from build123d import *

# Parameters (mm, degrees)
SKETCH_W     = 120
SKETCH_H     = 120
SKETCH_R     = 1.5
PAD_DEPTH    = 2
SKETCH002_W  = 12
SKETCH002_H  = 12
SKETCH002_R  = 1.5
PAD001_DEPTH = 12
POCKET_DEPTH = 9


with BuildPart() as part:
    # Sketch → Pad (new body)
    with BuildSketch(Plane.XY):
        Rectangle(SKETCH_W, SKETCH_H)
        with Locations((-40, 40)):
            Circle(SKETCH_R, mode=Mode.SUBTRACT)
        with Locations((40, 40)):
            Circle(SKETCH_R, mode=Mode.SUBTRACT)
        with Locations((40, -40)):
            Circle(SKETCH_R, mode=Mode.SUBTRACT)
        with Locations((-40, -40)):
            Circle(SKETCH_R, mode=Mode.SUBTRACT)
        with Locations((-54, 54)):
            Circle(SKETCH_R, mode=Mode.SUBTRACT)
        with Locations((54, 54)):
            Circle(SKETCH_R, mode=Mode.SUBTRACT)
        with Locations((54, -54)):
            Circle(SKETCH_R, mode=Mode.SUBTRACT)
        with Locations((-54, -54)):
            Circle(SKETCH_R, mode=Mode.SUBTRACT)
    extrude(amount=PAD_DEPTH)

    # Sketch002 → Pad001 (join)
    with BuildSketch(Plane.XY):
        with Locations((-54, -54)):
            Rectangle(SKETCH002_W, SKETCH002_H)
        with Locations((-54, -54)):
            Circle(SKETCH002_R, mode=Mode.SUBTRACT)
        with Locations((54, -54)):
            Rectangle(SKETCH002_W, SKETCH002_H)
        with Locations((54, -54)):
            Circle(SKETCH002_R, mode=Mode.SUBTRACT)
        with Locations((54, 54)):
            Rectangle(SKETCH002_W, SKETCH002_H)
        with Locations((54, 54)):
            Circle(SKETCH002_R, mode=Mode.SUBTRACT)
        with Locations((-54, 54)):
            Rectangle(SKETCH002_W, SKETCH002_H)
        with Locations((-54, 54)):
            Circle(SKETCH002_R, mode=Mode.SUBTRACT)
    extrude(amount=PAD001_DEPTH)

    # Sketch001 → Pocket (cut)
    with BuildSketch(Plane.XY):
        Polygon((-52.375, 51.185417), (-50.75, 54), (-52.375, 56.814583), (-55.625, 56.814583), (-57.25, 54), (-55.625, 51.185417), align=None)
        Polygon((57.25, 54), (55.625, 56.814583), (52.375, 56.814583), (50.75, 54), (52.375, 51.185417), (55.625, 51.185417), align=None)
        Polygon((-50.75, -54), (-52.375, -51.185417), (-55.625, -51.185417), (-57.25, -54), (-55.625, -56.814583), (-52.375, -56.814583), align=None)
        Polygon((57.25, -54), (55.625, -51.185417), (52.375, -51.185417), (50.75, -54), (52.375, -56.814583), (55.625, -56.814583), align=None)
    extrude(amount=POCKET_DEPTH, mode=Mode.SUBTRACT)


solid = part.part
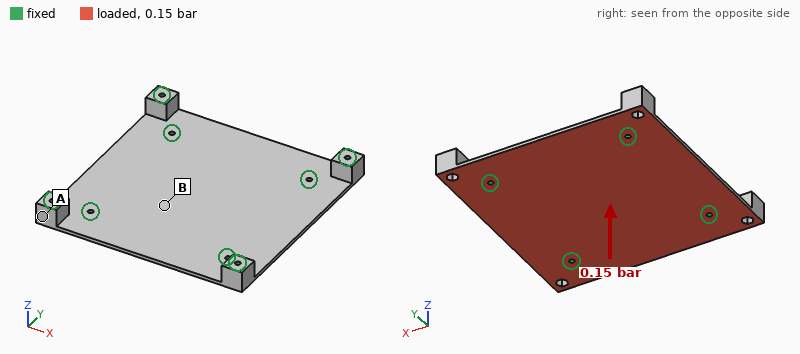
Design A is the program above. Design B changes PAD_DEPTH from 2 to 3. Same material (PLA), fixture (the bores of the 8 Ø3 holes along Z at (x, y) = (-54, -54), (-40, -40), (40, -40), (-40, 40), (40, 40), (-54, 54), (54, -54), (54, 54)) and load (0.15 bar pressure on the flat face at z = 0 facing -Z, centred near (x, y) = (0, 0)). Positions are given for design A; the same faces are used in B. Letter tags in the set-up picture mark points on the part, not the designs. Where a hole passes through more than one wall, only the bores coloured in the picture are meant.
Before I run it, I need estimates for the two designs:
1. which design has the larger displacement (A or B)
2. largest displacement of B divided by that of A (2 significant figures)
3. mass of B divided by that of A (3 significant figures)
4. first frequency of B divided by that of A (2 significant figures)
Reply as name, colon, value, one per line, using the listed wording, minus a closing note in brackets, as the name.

which design has the larger displacement: A
largest displacement of B divided by that of A: 0.31
mass of B divided by that of A: 1.41
first frequency of B divided by that of A: 1.5
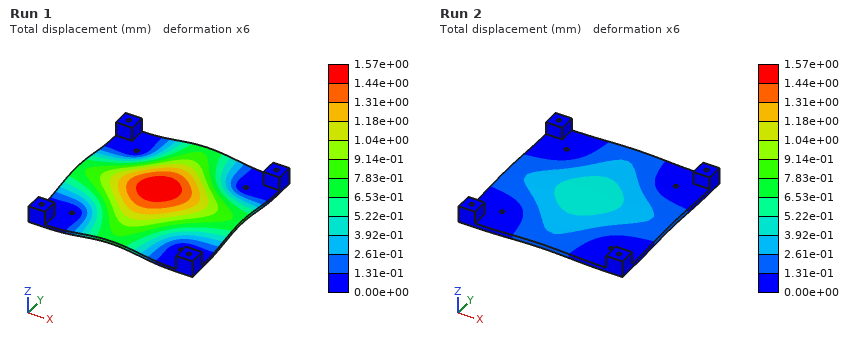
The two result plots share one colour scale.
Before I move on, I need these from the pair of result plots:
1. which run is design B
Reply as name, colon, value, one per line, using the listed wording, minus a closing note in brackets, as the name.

which run is design B: Run 2
